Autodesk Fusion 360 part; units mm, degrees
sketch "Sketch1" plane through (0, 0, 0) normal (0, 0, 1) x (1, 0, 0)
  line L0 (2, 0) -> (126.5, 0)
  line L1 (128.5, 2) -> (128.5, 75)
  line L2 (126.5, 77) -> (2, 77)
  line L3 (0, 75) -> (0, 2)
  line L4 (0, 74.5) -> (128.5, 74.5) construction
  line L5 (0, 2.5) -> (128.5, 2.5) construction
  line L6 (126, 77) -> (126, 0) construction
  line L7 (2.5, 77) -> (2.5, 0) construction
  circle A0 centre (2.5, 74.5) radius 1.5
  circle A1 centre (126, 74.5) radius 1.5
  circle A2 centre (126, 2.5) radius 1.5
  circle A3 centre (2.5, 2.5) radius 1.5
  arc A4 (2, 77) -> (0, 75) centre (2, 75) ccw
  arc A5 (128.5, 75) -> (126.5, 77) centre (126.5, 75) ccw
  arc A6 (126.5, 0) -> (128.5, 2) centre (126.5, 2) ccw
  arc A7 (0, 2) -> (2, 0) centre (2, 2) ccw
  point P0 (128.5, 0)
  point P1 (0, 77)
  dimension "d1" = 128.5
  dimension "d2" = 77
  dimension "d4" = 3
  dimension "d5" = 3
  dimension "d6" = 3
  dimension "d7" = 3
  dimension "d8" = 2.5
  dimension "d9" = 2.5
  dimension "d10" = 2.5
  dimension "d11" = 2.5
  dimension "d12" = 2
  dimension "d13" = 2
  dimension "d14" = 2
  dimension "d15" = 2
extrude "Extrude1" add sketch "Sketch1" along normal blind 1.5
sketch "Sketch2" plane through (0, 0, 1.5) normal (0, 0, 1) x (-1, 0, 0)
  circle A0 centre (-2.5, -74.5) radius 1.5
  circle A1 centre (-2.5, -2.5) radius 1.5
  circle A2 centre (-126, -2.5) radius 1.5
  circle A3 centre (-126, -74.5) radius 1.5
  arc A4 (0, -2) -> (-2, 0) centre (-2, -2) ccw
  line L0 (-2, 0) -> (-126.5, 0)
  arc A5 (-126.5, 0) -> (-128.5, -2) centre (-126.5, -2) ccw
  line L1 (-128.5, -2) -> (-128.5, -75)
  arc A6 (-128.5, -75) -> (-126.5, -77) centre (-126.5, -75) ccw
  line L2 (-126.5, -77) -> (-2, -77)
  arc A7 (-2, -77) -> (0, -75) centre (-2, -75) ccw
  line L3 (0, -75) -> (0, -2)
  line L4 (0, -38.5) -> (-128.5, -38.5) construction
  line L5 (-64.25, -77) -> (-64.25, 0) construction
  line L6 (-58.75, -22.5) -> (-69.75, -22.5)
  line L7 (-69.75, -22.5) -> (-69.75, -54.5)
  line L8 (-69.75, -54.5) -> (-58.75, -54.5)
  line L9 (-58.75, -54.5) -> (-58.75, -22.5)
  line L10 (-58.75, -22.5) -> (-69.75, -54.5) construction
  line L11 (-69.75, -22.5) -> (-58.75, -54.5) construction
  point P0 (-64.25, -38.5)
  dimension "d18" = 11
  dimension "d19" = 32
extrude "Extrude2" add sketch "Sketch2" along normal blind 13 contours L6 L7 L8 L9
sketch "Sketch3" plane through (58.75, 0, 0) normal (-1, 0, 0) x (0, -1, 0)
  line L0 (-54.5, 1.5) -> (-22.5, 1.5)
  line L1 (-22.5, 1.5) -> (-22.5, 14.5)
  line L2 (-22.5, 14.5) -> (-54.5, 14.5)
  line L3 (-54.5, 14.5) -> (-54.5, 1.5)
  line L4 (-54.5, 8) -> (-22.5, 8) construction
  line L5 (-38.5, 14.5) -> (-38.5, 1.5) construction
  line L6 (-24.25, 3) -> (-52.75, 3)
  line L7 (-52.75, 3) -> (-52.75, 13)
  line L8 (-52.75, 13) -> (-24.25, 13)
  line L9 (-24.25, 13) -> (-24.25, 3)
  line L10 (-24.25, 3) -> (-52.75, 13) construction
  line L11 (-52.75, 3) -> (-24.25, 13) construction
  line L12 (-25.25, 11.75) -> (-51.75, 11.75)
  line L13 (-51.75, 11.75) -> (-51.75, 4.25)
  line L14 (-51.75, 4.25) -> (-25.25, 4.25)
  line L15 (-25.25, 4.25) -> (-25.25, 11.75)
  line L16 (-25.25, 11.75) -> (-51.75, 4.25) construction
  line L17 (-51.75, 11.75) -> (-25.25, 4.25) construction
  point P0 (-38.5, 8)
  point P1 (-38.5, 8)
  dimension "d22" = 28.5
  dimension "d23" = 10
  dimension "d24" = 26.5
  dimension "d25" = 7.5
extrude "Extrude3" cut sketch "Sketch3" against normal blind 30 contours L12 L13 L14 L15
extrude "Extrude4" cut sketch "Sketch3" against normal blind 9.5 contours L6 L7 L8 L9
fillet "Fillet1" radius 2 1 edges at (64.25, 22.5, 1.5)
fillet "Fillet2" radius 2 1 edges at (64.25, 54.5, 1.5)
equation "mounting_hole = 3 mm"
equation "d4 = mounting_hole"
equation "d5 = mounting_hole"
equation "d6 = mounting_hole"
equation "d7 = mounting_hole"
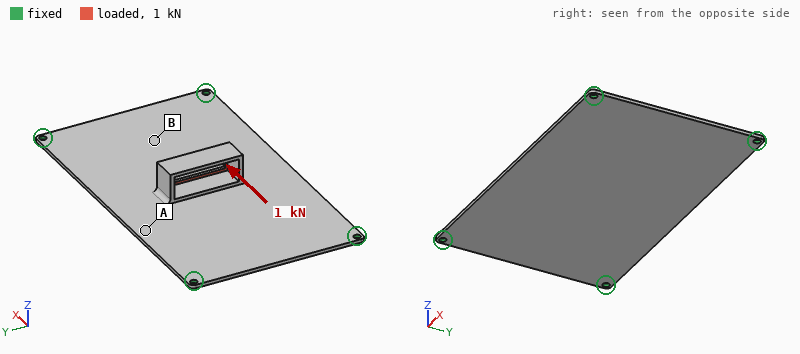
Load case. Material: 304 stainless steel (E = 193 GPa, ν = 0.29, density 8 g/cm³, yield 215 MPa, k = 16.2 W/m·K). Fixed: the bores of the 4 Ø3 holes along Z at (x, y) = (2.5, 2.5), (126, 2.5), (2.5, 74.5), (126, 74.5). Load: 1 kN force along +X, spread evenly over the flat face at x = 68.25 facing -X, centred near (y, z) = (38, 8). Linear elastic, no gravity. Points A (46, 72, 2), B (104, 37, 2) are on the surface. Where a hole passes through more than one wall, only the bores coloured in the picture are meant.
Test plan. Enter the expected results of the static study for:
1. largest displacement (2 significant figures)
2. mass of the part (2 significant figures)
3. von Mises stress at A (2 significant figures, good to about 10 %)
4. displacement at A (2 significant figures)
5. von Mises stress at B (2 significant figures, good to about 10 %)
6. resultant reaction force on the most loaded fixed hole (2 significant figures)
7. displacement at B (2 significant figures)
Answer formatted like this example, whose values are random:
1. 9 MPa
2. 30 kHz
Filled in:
1. 0.20 mm
2. 130 g
3. 68 MPa
4. 0.12 mm
5. 30 MPa
6. 280 N
7. 0.14 mm
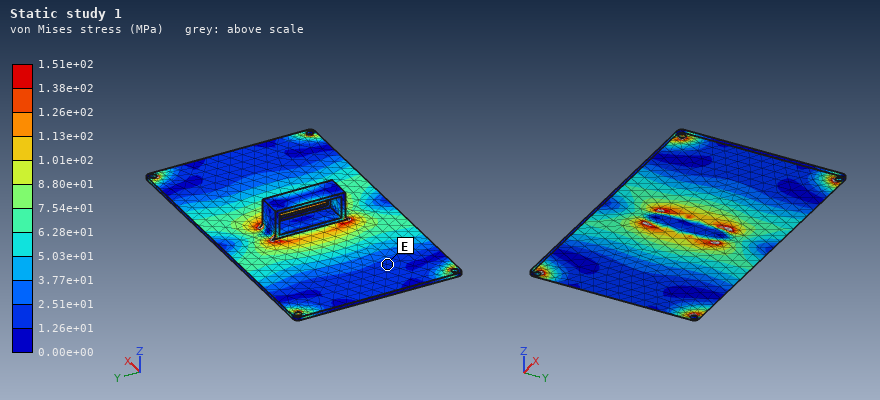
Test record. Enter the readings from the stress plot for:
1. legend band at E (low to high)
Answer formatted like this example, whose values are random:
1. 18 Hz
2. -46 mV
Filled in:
1. 1.26e+01 to 2.51e+01 MPa
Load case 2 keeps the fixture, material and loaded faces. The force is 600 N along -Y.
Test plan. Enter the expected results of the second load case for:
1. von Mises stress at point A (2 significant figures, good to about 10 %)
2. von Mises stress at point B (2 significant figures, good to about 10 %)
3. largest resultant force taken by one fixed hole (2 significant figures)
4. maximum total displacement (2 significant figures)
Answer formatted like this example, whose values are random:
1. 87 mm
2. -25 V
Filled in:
1. 37 MPa
2. 48 MPa
3. 210 N
4. 0.35 mm
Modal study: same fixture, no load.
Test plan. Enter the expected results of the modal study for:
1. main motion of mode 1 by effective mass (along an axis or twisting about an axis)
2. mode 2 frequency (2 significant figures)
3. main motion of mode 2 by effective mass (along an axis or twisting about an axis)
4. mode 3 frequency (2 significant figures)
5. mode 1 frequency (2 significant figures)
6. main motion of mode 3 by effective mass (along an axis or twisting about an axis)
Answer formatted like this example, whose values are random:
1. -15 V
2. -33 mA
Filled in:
1. along Z
2. 670 Hz
3. twisting about X
4. 990 Hz
5. 350 Hz
6. twisting about Y
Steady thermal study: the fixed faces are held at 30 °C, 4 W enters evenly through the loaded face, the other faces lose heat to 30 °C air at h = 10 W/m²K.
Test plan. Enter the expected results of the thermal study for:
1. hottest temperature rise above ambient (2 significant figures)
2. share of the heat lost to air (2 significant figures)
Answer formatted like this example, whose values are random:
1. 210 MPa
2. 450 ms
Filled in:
1. 77 K
2. 85 %
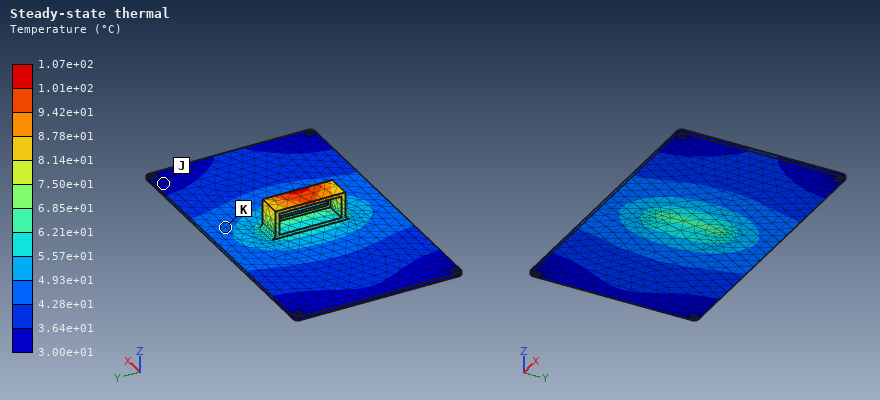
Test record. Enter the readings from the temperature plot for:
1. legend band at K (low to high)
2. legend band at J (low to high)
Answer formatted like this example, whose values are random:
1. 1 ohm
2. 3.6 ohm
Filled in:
1. 4.28e+01 to 4.93e+01 °C
2. 3.00e+01 to 3.64e+01 °C
